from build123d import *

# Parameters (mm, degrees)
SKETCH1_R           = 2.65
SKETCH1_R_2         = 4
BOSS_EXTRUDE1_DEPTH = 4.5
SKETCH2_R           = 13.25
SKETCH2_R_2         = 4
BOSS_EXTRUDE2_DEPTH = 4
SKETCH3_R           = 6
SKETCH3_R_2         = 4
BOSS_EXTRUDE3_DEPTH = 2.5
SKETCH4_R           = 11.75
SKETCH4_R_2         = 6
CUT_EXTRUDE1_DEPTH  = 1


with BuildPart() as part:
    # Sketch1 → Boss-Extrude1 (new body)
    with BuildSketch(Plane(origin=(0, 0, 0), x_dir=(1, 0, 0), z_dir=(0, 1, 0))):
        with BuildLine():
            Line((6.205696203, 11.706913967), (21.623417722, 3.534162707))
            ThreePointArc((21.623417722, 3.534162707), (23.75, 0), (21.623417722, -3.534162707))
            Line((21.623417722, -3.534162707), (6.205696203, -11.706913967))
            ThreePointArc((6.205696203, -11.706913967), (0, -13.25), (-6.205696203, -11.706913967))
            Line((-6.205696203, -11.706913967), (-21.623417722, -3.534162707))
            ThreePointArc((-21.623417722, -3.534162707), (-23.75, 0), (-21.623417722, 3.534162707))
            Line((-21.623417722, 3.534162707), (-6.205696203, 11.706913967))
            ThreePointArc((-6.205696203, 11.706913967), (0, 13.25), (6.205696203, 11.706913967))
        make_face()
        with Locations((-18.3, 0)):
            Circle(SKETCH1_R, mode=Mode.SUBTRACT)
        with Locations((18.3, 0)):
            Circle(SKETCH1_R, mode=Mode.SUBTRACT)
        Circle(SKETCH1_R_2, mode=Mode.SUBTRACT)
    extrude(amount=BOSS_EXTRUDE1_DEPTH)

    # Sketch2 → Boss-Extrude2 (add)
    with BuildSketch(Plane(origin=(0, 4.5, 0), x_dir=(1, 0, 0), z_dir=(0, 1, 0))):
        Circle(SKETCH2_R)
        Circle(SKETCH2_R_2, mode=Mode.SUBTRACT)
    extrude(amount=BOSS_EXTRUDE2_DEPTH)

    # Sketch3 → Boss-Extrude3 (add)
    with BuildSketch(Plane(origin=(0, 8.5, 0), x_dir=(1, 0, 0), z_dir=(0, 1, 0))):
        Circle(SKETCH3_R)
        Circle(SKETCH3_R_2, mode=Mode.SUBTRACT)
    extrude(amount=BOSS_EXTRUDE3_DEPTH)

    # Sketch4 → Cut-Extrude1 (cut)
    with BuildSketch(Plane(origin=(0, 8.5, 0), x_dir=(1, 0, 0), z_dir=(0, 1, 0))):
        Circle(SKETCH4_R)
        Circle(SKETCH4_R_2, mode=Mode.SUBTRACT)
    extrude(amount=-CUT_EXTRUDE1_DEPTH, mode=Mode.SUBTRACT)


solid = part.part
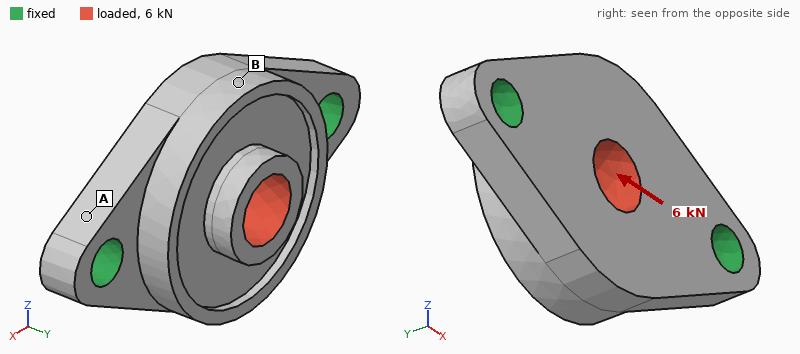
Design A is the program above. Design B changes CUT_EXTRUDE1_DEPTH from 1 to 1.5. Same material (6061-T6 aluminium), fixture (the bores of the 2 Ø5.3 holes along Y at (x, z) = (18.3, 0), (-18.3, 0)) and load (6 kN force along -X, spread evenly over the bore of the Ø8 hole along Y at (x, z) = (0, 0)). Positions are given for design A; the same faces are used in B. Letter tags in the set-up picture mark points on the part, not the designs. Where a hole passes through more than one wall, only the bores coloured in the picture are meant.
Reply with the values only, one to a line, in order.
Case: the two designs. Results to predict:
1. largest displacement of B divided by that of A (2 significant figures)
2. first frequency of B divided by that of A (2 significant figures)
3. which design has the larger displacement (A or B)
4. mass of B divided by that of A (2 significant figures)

1.1
1.0
B
0.97
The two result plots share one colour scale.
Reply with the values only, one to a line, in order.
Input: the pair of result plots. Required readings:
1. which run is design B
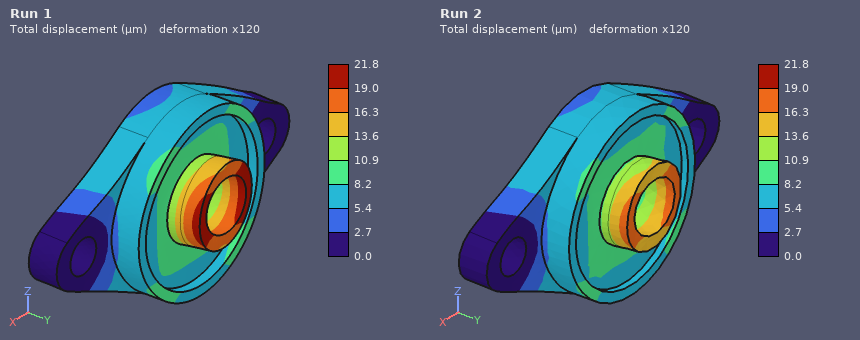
Run 1
